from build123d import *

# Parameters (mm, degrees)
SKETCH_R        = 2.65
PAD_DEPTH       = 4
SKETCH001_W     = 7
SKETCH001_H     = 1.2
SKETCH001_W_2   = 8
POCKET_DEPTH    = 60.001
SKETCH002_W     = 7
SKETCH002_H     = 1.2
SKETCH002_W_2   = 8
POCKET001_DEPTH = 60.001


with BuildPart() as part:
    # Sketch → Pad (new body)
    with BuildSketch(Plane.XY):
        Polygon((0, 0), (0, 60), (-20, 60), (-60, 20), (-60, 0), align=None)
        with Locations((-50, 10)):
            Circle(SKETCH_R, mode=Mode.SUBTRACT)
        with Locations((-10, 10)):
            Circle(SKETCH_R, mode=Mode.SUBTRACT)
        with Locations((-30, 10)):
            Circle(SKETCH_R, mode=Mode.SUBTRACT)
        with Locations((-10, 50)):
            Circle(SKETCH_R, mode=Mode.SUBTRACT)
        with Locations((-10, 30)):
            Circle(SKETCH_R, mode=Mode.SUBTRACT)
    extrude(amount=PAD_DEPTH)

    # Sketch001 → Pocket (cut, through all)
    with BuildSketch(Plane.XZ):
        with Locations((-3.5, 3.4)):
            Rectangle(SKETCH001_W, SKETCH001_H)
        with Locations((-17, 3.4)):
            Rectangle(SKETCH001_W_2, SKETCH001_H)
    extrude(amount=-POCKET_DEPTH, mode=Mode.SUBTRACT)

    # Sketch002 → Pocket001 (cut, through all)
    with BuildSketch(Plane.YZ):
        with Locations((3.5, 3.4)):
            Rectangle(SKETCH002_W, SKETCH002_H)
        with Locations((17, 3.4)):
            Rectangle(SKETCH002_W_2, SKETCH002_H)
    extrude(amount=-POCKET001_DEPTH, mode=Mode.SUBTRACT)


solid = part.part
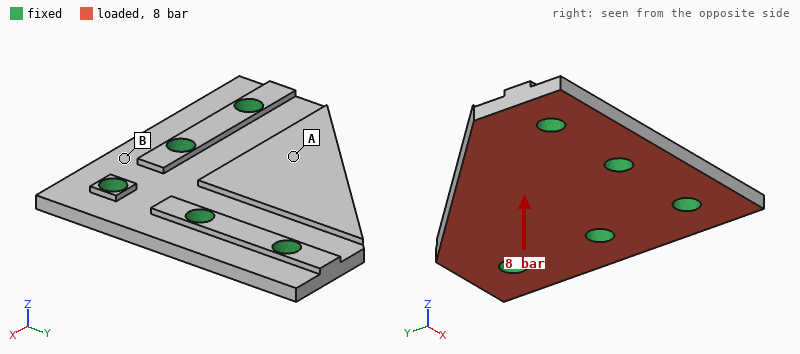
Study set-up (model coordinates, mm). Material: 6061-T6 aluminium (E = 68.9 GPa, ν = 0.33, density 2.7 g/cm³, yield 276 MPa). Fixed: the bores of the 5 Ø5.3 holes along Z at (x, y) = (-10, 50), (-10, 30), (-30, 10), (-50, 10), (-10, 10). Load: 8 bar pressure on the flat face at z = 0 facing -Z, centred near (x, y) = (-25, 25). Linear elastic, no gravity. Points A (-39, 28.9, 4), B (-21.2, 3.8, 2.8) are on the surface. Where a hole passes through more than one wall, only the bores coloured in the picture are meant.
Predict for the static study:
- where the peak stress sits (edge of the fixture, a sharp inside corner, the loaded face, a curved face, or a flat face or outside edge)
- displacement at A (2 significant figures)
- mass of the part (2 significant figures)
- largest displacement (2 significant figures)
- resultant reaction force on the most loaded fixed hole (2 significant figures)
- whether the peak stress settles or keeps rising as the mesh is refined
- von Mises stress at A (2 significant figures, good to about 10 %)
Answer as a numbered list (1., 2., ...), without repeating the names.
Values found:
1. edge of the fixture
2. 0.061 mm
3. 24 g
4. 0.10 mm
5. 540 N
6. keeps rising
7. 31 MPa
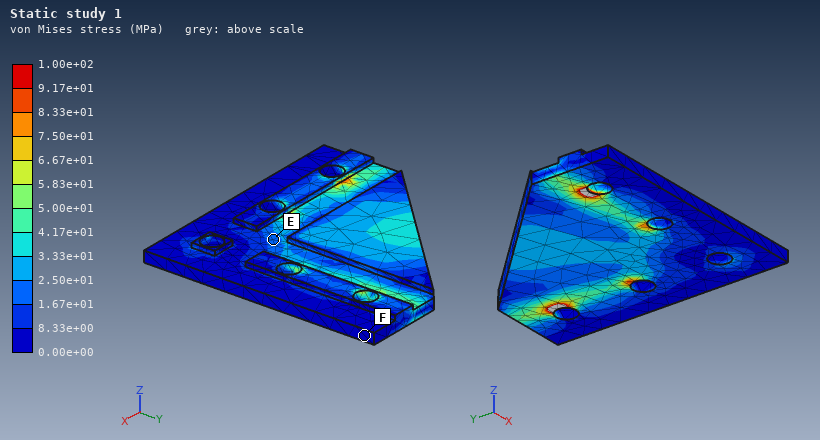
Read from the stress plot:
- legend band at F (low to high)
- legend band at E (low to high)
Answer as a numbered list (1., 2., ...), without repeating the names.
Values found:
1. 0.00e+00 to 8.33e+00 MPa
2. 1.67e+01 to 2.50e+01 MPa
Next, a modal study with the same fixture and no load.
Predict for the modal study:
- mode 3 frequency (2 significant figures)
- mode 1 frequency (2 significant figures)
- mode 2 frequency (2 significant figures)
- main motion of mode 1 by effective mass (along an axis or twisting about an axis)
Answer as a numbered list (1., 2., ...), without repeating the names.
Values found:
1. 19 kHz
2. 5800 Hz
3. 13 kHz
4. along Z
